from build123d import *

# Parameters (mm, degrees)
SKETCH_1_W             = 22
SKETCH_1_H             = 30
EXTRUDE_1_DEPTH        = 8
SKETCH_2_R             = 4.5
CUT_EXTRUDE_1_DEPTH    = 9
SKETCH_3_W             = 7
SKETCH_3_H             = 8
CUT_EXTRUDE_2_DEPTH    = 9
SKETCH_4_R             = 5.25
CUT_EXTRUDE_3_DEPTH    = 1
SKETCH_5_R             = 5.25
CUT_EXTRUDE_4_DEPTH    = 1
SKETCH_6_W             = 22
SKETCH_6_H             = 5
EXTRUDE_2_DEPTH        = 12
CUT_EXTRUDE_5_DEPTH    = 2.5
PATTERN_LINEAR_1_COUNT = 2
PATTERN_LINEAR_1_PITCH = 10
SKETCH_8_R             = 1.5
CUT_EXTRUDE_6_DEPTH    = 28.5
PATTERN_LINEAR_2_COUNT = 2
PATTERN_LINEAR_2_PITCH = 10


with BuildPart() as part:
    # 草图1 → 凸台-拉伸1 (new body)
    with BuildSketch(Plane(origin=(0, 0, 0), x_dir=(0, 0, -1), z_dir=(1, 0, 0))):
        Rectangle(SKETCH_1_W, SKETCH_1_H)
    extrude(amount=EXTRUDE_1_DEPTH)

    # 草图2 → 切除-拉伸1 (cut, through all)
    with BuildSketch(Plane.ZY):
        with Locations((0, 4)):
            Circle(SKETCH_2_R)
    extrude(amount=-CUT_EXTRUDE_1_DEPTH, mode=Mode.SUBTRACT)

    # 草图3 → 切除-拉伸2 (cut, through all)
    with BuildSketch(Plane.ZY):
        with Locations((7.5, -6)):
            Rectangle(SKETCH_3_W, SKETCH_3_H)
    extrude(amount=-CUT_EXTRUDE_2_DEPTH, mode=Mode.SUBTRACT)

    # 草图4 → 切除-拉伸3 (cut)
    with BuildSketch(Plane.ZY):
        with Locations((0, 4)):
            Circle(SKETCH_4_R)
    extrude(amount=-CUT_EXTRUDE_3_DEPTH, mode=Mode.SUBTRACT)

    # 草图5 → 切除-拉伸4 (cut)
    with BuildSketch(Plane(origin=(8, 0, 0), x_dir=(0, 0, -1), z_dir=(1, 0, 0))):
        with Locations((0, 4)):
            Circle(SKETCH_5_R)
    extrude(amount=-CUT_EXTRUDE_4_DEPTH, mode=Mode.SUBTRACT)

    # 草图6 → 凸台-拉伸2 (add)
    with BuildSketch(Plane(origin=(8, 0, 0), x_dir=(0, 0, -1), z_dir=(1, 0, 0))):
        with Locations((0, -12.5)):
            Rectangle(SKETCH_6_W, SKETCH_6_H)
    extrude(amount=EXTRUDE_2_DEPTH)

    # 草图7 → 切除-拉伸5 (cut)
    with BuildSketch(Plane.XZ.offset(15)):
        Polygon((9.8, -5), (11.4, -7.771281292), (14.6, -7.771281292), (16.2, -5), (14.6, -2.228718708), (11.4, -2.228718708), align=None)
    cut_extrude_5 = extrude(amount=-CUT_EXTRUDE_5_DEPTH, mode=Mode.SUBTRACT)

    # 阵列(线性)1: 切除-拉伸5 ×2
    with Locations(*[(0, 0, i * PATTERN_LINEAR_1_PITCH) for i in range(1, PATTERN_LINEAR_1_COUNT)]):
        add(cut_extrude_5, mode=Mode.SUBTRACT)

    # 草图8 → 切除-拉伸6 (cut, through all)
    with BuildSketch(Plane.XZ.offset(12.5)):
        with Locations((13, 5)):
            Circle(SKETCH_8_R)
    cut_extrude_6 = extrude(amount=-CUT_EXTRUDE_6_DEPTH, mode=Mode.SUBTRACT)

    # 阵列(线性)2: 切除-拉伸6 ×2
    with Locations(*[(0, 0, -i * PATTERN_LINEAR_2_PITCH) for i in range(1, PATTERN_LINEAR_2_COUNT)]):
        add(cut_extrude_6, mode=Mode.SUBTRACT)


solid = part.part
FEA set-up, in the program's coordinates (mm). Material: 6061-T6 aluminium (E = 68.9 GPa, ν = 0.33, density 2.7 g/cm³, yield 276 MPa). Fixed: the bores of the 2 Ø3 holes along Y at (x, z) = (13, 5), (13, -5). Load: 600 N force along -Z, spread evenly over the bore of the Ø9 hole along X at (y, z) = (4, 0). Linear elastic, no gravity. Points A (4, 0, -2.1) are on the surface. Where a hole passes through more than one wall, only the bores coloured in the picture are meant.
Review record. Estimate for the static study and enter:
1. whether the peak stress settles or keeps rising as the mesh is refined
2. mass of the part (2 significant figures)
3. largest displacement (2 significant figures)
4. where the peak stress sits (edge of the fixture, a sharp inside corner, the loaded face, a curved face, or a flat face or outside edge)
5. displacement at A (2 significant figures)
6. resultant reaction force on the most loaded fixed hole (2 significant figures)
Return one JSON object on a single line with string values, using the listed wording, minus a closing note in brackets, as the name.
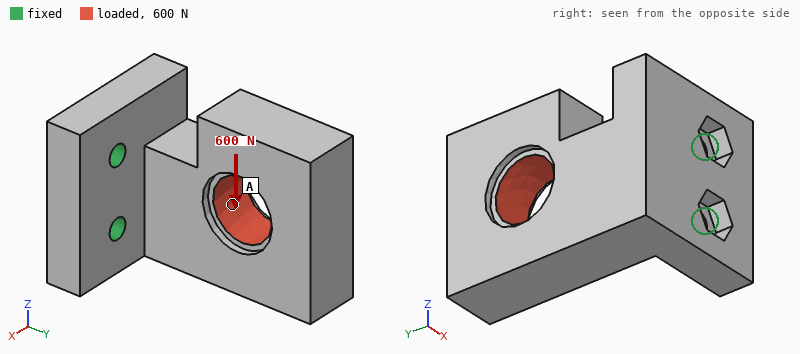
{"whether the peak stress settles or keeps rising as the mesh is refined": "keeps rising", "mass of the part": "15 g", "largest displacement": "0.10 mm", "where the peak stress sits": "edge of the fixture", "displacement at A": "0.040 mm", "resultant reaction force on the most loaded fixed hole": "930 N"}
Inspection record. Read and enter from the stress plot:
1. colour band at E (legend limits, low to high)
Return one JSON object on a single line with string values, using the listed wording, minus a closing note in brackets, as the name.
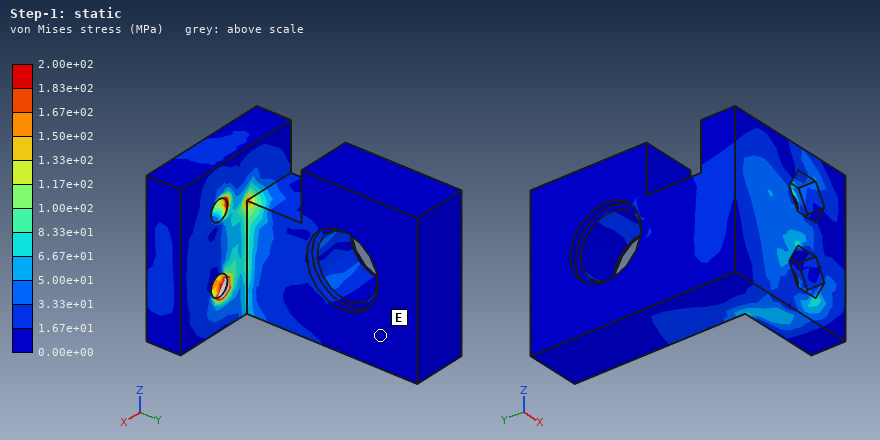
{"colour band at E": "0.00e+00 to 1.67e+01 MPa"}
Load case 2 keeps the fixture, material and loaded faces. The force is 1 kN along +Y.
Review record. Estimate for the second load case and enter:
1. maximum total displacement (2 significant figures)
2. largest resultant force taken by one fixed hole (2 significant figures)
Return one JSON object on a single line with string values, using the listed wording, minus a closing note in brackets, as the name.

{"maximum total displacement": "0.19 mm", "largest resultant force taken by one fixed hole": "510 N"}
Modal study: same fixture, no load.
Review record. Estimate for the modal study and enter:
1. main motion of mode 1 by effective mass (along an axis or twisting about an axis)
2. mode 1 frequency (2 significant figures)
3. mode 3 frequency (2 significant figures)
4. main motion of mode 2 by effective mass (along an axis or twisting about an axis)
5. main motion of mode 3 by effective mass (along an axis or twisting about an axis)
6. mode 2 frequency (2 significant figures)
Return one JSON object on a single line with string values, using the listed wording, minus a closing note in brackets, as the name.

{"main motion of mode 1 by effective mass": "along X", "mode 1 frequency": "2700 Hz", "mode 3 frequency": "11 kHz", "main motion of mode 2 by effective mass": "along Z", "main motion of mode 3 by effective mass": "along Y", "mode 2 frequency": "4800 Hz"}
